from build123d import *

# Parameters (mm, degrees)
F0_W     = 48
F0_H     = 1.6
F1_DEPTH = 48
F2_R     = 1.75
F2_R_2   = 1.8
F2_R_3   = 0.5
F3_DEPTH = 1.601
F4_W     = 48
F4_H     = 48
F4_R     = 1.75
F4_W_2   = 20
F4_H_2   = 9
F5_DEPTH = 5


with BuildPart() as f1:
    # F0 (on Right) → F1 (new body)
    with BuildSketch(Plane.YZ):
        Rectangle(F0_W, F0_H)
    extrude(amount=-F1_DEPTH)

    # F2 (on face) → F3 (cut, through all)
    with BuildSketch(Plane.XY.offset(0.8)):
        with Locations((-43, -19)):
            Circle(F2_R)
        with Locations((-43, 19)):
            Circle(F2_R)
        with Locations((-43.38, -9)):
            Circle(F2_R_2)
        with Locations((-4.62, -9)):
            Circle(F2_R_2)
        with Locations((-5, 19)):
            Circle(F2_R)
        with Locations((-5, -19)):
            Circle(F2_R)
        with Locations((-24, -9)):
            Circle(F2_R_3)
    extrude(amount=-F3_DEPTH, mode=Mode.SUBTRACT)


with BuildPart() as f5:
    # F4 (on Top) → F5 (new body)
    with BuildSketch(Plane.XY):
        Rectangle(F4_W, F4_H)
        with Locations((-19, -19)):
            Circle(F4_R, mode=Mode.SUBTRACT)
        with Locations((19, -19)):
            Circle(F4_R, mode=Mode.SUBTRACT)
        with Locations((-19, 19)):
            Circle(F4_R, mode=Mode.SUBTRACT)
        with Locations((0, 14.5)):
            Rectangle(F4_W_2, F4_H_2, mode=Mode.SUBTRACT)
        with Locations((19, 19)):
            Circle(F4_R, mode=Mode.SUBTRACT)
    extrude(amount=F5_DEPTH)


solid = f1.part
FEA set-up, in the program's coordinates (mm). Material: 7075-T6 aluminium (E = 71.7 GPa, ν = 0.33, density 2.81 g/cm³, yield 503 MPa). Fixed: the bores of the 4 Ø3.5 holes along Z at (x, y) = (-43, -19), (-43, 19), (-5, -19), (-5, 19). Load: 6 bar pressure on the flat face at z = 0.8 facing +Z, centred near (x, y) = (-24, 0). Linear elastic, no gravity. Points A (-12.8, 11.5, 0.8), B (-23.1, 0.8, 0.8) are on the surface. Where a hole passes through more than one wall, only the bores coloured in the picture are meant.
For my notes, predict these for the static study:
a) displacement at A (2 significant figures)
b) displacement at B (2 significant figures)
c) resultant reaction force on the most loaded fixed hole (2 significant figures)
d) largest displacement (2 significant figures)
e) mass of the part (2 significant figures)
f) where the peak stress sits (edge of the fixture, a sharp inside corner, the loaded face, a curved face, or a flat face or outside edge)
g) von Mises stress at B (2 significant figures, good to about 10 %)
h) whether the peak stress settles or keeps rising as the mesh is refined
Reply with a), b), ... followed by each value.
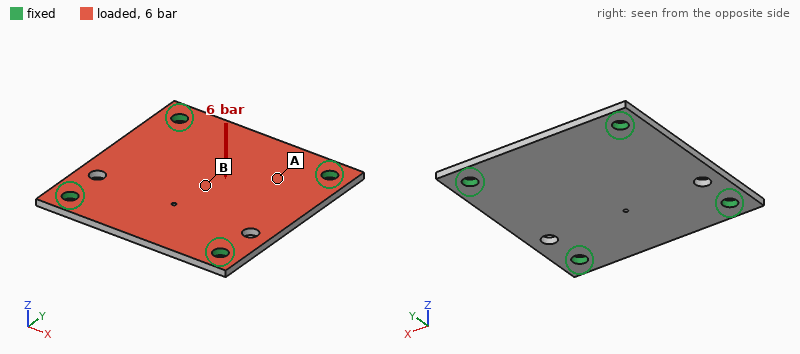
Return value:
a) 0.14 mm
b) 0.28 mm
c) 340 N
d) 0.28 mm
e) 10 g
f) edge of the fixture
g) 98 MPa
h) keeps rising
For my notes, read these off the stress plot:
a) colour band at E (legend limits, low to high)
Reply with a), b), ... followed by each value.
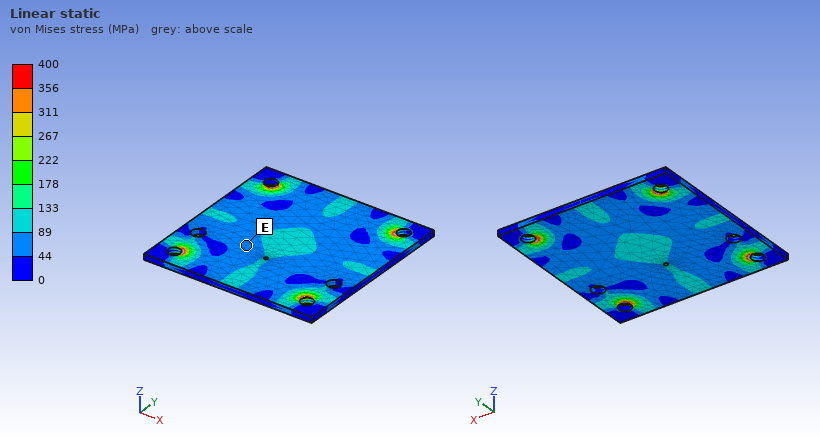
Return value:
a) 44 to 89 MPa
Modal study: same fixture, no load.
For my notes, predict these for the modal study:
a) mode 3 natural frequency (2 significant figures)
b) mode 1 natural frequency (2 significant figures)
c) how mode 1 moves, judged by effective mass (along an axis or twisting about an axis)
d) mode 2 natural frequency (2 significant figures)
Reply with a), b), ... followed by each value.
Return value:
a) 6900 Hz
b) 4300 Hz
c) along Z
d) 6900 Hz
